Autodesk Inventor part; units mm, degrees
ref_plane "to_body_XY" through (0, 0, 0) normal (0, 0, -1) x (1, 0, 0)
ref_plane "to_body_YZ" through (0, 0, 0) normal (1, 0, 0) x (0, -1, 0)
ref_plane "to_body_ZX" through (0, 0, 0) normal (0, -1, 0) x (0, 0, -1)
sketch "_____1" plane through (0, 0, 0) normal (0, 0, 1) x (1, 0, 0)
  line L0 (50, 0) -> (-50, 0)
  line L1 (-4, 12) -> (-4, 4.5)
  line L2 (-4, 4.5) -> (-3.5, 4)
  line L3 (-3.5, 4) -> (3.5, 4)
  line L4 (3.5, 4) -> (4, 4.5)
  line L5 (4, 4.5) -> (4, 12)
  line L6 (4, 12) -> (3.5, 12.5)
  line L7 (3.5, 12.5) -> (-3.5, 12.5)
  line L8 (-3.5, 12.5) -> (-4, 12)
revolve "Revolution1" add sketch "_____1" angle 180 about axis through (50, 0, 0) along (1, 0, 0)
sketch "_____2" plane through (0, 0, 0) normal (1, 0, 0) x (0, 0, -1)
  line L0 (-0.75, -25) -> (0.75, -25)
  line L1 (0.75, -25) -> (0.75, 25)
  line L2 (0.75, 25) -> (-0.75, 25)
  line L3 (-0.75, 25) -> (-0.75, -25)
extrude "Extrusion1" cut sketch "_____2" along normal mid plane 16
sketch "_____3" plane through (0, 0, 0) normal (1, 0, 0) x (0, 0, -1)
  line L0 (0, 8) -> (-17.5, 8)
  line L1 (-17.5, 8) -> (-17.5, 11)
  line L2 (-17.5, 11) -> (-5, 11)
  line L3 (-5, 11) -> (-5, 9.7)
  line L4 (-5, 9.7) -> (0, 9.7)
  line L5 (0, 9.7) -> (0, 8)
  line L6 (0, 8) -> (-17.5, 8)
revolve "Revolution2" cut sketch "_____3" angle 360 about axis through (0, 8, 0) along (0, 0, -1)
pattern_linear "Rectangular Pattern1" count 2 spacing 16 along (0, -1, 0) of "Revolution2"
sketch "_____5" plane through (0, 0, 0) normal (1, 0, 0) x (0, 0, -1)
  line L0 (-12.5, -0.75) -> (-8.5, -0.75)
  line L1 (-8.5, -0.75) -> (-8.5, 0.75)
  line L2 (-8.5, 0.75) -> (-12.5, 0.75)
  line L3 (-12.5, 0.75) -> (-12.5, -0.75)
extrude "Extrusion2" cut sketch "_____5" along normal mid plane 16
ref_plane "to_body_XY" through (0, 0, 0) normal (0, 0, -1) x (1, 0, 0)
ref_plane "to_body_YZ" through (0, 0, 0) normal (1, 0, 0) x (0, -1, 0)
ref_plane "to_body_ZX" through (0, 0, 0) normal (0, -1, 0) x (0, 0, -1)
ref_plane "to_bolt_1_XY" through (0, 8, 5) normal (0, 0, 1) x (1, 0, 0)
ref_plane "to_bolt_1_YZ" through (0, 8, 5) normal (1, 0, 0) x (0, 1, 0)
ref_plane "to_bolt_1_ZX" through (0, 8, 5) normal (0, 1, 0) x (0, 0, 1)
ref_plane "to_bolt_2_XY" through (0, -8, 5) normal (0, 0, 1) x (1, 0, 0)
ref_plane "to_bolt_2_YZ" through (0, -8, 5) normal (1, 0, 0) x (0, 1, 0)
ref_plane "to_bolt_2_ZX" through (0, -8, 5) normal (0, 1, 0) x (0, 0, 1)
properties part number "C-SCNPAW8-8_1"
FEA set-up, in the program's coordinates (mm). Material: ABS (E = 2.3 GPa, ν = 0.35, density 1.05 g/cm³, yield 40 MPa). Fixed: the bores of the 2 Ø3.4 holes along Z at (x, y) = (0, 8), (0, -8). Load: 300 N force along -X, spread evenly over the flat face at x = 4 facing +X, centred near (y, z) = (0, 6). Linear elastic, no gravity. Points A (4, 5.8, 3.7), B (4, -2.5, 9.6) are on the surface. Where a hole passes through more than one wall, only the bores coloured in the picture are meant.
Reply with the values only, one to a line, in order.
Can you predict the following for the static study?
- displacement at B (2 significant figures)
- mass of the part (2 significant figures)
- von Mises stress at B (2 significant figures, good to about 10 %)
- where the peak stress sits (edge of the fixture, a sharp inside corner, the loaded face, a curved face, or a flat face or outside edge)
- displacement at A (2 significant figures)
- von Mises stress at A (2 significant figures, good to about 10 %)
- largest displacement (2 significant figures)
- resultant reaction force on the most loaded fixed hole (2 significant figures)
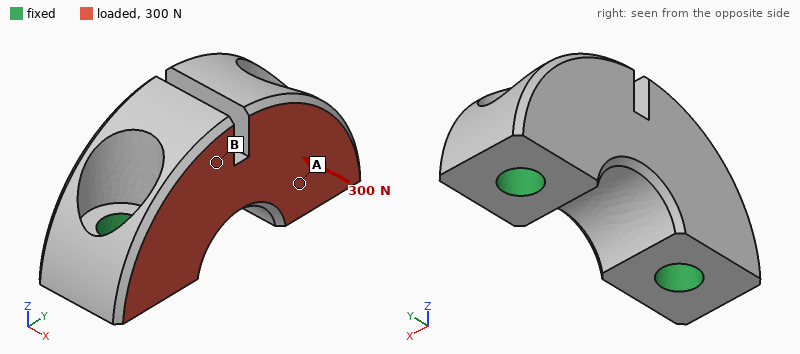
76 µm
1.3 g
2.2 MPa
edge of the fixture
24 µm
10 MPa
93 µm
150 N
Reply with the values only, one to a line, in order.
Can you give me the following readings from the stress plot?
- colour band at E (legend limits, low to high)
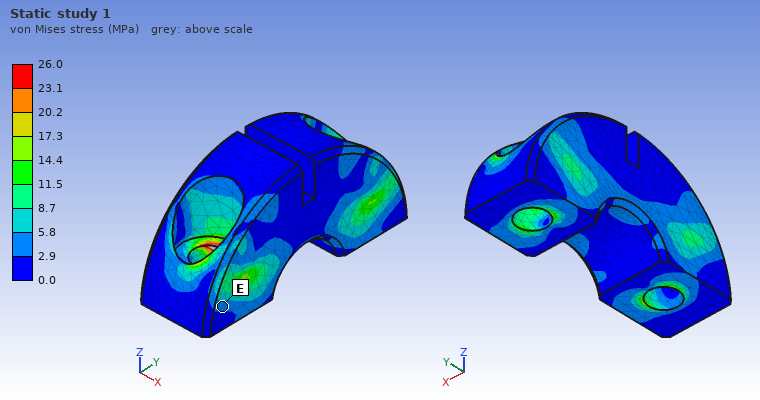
2.9 to 5.8 MPa
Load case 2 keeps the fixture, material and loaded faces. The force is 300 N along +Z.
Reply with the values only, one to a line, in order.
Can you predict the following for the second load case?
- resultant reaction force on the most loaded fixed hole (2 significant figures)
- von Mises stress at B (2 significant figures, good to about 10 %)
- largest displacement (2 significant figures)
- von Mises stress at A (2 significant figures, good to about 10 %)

160 N
3.6 MPa
90 µm
9.7 MPa
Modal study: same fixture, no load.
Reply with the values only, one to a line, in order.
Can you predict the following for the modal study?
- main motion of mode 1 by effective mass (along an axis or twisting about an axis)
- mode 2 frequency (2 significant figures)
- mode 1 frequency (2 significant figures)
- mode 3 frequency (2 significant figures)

along X
18 kHz
9200 Hz
18 kHz
